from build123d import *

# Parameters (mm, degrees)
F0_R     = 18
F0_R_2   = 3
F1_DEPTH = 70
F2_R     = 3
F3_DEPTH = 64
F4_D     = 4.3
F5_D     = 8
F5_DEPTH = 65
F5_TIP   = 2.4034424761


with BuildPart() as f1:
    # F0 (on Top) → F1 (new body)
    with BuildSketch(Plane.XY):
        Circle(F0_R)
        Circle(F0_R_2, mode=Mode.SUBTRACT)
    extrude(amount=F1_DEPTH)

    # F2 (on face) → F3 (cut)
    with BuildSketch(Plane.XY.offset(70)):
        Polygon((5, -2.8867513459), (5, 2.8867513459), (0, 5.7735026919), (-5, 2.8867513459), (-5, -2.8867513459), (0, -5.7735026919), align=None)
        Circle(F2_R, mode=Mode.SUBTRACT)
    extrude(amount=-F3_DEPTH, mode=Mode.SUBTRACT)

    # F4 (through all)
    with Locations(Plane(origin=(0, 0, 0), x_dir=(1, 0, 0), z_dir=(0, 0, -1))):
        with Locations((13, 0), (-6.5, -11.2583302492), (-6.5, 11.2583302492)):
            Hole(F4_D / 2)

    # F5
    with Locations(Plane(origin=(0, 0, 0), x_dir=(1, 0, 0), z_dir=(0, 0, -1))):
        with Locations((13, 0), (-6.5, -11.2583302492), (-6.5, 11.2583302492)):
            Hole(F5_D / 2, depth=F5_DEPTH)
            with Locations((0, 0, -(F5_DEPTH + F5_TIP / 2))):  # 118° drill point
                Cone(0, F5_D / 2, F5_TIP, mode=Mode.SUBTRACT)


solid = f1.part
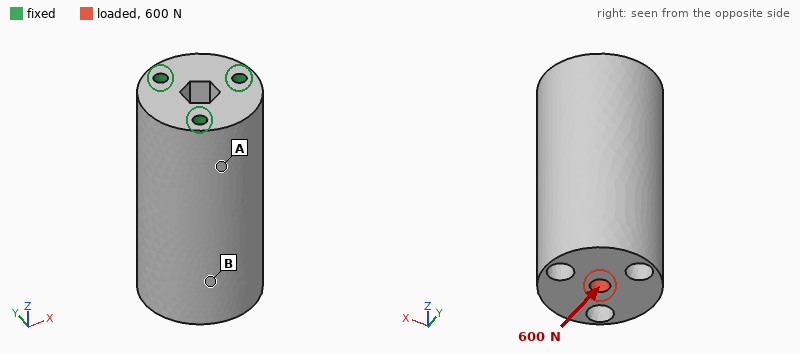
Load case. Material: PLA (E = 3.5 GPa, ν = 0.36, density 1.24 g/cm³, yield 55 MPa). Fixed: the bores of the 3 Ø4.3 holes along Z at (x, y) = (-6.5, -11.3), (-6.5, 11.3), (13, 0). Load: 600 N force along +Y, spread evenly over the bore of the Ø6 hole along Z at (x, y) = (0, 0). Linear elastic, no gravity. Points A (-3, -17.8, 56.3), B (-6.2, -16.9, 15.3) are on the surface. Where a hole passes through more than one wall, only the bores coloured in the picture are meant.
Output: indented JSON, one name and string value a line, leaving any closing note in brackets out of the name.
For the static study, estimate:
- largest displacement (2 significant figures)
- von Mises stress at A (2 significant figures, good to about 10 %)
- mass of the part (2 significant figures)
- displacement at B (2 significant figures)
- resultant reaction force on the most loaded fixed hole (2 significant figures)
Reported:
{
  "largest displacement": "0.77 mm",
  "von Mises stress at A": "12 MPa",
  "mass of the part": "69 g",
  "displacement at B": "0.58 mm",
  "resultant reaction force on the most loaded fixed hole": "1.6 kN"
}
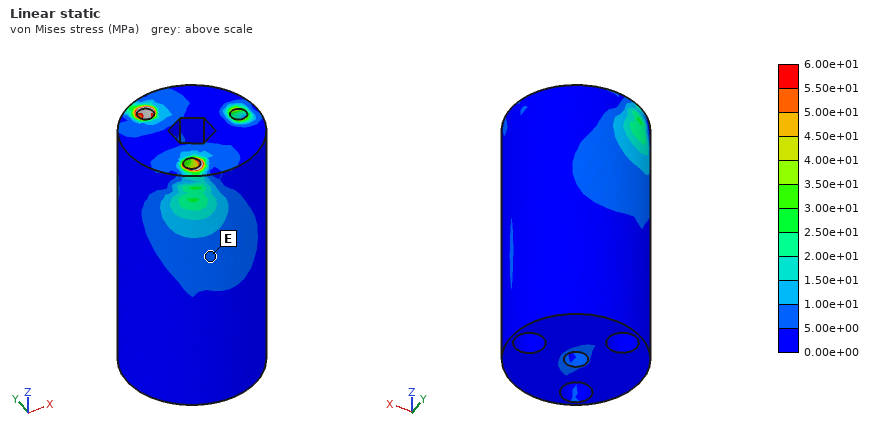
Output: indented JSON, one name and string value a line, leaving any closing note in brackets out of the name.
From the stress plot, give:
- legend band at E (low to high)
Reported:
{
  "legend band at E": "5.00e+00 to 1.00e+01 MPa"
}
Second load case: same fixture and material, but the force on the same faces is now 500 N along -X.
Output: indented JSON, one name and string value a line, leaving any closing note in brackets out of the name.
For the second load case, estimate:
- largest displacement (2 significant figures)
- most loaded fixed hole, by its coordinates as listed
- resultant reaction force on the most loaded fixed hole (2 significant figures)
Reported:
{
  "largest displacement": "0.64 mm",
  "most loaded fixed hole, by its coordinates as listed": "(13, 0)",
  "resultant reaction force on the most loaded fixed hole": "1.5 kN"
}
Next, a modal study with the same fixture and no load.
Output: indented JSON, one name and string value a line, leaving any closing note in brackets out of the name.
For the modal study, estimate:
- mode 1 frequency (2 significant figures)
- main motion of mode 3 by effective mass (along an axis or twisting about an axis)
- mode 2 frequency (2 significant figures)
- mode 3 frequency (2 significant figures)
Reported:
{
  "mode 1 frequency": "950 Hz",
  "main motion of mode 3 by effective mass": "twisting about Z",
  "mode 2 frequency": "950 Hz",
  "mode 3 frequency": "3100 Hz"
}
